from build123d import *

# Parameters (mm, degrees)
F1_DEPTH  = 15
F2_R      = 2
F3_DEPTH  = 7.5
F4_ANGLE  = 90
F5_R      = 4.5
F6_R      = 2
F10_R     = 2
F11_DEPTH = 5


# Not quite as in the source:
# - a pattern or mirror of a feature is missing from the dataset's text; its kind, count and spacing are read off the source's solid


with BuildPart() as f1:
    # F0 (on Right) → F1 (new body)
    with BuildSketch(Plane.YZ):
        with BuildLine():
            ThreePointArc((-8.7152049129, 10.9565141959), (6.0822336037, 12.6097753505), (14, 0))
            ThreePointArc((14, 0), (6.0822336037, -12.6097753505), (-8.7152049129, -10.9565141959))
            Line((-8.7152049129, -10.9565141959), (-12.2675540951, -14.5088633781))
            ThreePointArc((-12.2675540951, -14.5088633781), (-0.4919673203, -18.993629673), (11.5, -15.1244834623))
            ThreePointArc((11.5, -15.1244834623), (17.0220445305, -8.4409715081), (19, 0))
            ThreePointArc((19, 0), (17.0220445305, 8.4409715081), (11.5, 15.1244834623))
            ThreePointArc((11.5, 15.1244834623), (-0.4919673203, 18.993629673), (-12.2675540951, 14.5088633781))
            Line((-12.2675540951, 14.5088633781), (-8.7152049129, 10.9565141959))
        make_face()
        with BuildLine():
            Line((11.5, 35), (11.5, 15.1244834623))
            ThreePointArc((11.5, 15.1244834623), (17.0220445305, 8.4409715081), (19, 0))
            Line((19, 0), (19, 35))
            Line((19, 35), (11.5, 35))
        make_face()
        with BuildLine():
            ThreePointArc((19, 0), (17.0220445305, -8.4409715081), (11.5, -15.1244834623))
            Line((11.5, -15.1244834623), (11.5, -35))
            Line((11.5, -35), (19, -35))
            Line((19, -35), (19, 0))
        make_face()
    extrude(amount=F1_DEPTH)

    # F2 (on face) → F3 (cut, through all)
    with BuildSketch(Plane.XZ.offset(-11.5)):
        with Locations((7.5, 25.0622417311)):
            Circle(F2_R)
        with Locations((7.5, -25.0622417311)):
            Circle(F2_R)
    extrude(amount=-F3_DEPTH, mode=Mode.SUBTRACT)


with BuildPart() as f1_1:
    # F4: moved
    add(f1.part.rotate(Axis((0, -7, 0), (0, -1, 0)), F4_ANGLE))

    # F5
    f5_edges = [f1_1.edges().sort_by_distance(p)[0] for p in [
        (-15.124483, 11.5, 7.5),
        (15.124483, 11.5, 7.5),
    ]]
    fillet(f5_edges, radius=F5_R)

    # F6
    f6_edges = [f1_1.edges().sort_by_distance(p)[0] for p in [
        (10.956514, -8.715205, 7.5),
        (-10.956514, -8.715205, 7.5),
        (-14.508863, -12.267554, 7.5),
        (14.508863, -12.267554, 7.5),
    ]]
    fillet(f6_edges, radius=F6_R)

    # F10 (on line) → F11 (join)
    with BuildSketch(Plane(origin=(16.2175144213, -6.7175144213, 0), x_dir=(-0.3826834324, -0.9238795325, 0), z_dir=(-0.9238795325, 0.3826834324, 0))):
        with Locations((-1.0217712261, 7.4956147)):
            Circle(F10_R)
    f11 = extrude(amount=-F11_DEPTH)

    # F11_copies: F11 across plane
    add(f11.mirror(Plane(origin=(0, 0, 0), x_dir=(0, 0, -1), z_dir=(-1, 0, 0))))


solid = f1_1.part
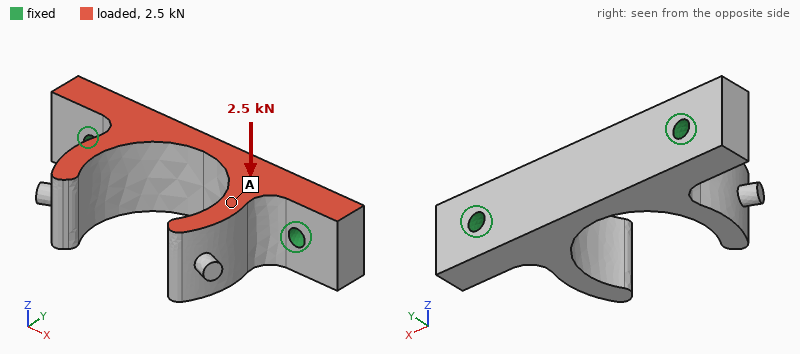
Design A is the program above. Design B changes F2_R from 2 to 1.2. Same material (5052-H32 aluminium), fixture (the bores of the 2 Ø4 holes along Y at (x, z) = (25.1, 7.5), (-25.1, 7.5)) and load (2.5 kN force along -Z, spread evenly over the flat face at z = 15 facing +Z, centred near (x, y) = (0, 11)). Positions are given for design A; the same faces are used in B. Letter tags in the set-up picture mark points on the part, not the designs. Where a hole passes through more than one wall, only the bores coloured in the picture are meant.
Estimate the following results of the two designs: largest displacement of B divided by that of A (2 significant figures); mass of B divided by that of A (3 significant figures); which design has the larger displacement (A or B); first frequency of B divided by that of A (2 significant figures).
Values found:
1.3
1.01
B
0.94
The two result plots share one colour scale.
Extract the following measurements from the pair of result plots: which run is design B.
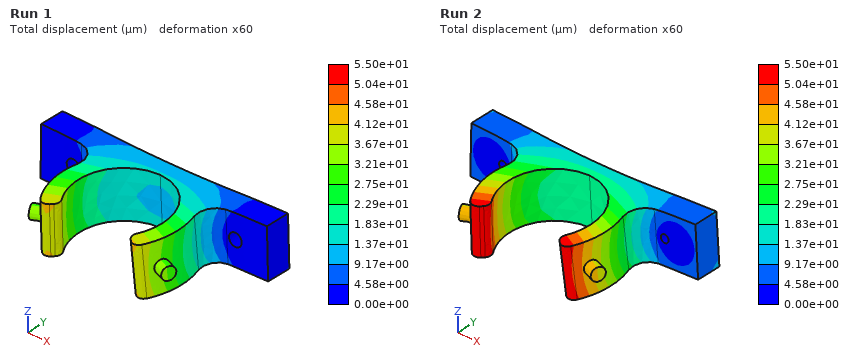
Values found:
Run 2
